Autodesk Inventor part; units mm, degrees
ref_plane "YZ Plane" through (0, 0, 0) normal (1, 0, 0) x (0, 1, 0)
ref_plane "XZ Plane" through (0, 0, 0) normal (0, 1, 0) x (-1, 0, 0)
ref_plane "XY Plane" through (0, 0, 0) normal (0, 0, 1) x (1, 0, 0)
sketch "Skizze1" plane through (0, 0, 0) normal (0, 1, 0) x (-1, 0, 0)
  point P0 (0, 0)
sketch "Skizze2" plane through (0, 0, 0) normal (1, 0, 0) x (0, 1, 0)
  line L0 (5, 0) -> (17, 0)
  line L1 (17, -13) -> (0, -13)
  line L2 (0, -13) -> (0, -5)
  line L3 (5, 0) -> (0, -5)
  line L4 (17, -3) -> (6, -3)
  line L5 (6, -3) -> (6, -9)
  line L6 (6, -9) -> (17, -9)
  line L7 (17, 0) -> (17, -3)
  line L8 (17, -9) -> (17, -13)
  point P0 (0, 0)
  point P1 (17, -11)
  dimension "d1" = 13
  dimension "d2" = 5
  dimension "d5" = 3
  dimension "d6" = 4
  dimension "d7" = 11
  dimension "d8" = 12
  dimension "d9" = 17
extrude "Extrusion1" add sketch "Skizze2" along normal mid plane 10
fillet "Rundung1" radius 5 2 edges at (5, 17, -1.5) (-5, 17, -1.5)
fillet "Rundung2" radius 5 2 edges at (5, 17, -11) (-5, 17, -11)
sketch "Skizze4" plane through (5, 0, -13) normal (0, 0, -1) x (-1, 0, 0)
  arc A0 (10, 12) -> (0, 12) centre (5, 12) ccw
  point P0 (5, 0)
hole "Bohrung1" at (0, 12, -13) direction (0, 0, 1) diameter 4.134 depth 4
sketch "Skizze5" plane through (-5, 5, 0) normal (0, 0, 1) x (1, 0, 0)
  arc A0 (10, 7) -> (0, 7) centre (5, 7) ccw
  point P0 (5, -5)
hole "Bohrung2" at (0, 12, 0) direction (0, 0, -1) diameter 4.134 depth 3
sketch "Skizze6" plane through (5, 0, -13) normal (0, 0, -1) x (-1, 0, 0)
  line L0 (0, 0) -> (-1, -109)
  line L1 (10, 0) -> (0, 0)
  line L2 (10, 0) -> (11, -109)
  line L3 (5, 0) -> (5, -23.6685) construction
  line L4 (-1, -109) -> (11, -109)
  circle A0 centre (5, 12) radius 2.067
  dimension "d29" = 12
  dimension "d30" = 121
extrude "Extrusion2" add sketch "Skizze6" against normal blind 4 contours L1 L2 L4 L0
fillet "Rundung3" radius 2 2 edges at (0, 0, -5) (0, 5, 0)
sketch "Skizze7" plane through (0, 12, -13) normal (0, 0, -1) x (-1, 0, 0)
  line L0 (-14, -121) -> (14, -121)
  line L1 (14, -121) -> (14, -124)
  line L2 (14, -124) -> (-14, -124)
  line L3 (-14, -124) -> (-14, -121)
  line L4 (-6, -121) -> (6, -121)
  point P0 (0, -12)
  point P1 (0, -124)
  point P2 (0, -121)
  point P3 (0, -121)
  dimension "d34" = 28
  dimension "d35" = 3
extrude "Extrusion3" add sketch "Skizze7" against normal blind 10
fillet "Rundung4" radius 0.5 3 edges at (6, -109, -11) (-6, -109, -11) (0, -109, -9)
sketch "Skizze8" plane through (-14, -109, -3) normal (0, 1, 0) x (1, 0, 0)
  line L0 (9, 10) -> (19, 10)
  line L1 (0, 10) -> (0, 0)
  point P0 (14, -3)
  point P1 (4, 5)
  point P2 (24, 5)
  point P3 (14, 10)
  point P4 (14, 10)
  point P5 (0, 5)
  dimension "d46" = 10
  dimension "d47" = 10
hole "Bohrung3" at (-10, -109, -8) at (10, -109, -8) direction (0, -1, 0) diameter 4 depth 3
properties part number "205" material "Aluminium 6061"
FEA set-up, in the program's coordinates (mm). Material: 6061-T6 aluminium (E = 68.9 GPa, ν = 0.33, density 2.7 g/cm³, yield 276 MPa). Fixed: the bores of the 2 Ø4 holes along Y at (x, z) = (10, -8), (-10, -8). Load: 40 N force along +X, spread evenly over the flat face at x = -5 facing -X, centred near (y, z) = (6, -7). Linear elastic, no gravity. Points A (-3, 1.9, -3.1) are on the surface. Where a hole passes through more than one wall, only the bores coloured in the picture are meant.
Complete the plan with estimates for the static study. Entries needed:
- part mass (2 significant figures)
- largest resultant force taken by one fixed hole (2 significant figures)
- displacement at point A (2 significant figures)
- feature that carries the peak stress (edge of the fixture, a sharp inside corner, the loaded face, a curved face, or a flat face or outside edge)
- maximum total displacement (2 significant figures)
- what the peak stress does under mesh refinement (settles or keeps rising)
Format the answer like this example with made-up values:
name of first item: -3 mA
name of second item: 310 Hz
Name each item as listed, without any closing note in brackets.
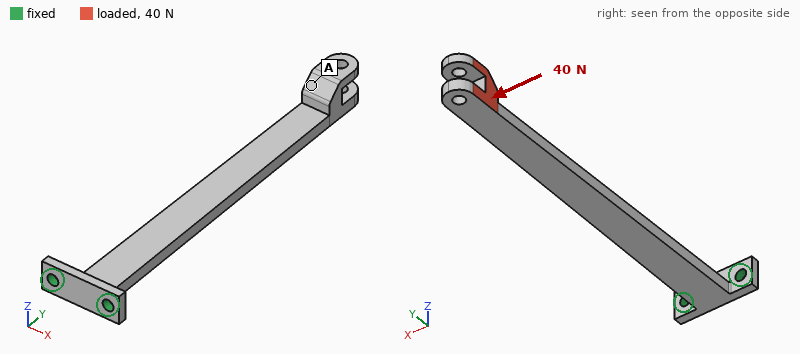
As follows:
part mass: 18 g
largest resultant force taken by one fixed hole: 320 N
displacement at point A: 0.69 mm
feature that carries the peak stress: a sharp inside corner
maximum total displacement: 0.84 mm
what the peak stress does under mesh refinement: keeps rising
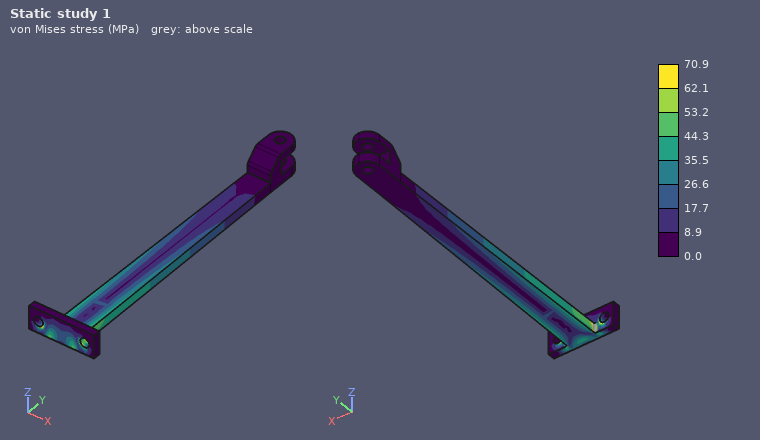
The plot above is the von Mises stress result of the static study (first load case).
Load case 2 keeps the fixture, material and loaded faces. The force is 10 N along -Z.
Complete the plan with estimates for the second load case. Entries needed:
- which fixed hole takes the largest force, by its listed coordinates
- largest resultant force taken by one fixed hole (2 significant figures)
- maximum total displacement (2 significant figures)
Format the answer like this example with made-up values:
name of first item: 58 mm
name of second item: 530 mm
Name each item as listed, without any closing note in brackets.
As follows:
which fixed hole takes the largest force, by its listed coordinates: (-10, -8)
largest resultant force taken by one fixed hole: 15 N
maximum total displacement: 1.6 mm
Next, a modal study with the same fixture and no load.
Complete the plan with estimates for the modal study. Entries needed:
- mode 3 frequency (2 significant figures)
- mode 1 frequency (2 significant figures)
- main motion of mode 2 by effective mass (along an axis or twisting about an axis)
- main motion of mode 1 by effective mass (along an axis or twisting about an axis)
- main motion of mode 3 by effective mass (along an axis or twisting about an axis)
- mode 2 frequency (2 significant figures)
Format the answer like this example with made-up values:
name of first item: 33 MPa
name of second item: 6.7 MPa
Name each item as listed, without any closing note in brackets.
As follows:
mode 3 frequency: 1100 Hz
mode 1 frequency: 170 Hz
main motion of mode 2 by effective mass: along X
main motion of mode 1 by effective mass: along Z
main motion of mode 3 by effective mass: along Z
mode 2 frequency: 490 Hz
